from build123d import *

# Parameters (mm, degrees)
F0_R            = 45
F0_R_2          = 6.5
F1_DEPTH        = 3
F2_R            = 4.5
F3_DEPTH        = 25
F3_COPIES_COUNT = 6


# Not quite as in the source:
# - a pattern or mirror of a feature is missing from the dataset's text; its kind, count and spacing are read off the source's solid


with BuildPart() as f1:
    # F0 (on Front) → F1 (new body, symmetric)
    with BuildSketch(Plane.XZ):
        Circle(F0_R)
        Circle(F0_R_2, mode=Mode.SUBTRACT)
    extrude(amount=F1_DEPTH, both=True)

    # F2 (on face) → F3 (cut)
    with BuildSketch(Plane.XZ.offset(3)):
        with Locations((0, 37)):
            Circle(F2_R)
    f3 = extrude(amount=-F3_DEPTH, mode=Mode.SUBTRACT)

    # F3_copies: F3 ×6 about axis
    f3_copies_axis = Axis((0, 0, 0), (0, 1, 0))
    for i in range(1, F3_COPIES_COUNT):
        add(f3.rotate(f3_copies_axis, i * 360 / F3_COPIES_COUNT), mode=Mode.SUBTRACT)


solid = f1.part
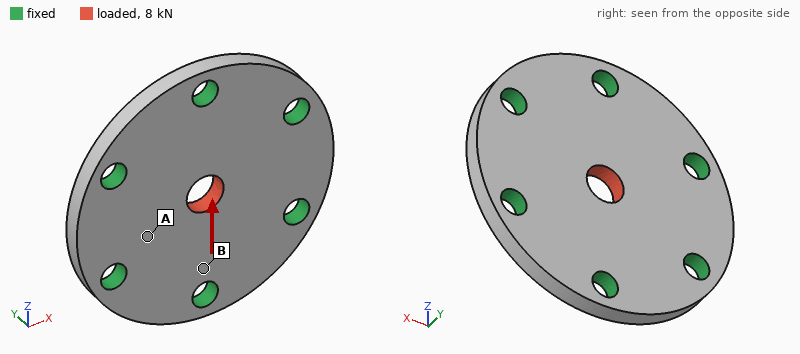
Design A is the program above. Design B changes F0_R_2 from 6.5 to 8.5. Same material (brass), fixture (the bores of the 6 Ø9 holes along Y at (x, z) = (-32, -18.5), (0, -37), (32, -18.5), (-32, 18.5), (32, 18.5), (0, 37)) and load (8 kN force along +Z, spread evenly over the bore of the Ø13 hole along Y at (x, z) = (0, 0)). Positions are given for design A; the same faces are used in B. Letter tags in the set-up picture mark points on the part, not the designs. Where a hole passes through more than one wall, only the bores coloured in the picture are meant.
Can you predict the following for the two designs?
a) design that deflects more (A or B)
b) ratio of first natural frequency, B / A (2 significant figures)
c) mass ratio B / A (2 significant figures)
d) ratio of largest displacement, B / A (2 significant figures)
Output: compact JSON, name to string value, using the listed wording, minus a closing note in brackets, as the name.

{"design that deflects more": "A", "ratio of first natural frequency, B / A": "1.0", "mass ratio B / A": "0.98", "ratio of largest displacement, B / A": "0.85"}
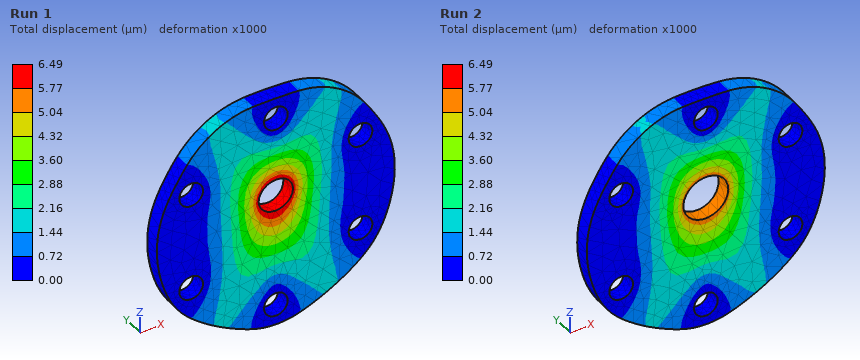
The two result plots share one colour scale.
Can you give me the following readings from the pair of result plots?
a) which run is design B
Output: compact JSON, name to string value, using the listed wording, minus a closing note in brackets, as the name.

{"which run is design B": "Run 2"}
